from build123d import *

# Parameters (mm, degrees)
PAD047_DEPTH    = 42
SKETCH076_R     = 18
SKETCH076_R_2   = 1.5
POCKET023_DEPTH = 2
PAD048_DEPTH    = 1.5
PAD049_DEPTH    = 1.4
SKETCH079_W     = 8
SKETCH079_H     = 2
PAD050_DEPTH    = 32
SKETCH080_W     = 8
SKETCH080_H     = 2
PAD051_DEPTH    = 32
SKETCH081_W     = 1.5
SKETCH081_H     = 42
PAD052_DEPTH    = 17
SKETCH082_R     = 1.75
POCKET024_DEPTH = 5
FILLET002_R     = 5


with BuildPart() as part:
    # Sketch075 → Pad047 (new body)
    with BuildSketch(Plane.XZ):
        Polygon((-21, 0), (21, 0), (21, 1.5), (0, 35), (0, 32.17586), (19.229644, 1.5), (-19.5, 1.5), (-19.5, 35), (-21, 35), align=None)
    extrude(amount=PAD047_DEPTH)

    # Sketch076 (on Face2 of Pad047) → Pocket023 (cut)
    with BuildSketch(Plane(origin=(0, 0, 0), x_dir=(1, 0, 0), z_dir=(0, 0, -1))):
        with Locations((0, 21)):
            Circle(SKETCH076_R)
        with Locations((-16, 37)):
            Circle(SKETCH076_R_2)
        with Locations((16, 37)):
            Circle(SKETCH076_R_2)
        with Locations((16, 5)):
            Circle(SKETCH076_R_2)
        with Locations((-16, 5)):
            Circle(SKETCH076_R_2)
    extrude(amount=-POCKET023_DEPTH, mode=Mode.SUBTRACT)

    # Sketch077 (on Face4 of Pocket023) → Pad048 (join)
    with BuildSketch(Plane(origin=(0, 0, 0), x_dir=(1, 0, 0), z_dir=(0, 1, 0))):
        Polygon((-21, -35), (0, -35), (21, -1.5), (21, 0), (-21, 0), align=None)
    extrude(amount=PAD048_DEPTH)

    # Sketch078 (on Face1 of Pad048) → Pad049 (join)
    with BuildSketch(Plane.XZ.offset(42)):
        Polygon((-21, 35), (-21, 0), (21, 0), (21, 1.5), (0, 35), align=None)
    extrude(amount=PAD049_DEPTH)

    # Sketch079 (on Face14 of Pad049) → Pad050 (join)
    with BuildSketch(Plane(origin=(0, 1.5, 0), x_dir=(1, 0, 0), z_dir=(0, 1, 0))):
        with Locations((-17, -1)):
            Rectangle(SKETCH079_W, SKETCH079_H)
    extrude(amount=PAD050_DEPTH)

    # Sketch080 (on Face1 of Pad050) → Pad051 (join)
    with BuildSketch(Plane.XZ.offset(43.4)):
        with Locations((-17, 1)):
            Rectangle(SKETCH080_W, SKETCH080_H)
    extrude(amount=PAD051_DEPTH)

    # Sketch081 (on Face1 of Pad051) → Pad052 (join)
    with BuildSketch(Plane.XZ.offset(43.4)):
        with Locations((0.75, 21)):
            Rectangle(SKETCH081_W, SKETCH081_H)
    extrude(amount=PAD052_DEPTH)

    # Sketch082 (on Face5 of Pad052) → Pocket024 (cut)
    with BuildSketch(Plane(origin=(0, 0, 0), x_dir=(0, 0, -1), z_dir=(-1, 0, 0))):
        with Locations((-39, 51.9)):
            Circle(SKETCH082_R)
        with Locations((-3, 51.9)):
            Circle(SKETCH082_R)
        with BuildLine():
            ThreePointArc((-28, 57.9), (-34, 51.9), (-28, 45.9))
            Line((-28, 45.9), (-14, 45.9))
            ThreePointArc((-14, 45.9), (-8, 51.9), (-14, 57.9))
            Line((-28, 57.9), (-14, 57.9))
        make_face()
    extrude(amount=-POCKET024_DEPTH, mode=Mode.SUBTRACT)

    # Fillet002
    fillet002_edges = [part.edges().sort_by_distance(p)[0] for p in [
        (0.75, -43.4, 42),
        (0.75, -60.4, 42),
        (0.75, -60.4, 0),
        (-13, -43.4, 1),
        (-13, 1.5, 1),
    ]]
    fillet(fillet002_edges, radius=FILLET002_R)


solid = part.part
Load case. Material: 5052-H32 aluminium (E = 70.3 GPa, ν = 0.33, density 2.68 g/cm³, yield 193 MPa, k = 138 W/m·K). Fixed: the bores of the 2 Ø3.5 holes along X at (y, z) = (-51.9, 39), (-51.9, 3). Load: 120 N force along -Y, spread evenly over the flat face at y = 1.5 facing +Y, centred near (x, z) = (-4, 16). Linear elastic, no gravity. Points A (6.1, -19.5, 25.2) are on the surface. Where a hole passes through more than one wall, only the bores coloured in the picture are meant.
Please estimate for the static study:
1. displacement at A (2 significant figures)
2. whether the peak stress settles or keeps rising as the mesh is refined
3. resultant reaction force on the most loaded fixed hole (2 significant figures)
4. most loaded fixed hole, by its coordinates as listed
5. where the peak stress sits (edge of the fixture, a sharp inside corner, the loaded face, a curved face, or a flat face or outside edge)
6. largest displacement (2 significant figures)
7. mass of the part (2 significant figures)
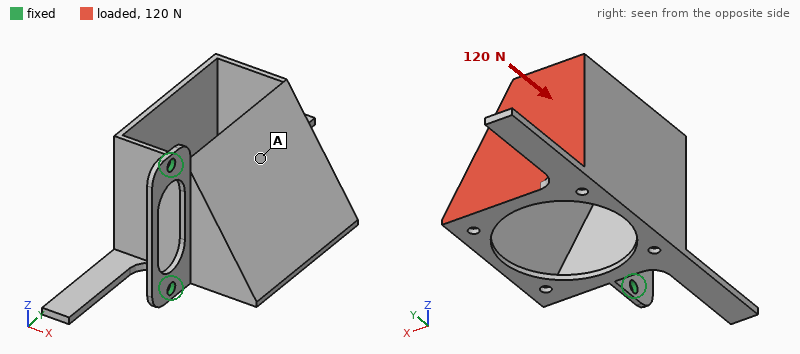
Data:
0.40 mm
keeps rising
73 N
(-51.9, 3)
edge of the fixture
1.3 mm
28 g
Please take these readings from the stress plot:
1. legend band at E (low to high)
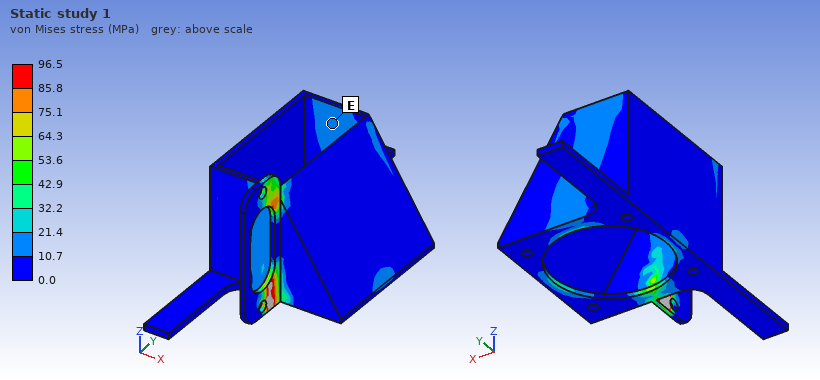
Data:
10.7 to 21.4 MPa
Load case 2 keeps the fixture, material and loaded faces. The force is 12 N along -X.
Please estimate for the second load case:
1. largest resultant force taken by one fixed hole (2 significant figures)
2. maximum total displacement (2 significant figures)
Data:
16 N
1.3 mm
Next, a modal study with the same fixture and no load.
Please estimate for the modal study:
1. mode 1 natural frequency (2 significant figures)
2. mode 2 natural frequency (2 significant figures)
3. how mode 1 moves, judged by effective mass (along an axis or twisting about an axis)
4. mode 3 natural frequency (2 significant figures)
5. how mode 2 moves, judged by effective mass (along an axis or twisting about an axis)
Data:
170 Hz
840 Hz
along X
1400 Hz
along Z
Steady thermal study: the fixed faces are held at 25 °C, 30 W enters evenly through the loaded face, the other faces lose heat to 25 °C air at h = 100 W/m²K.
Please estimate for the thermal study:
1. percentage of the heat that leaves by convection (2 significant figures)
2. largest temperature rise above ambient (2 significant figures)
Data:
91 %
50 K
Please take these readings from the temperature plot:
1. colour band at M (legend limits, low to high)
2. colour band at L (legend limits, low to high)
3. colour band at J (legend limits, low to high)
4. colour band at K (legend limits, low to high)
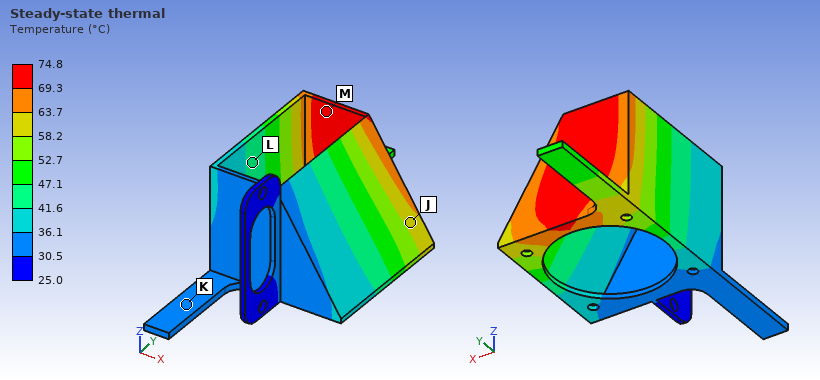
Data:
69.3 to 74.8 °C
41.6 to 47.1 °C
58.2 to 63.7 °C
30.5 to 36.1 °C
